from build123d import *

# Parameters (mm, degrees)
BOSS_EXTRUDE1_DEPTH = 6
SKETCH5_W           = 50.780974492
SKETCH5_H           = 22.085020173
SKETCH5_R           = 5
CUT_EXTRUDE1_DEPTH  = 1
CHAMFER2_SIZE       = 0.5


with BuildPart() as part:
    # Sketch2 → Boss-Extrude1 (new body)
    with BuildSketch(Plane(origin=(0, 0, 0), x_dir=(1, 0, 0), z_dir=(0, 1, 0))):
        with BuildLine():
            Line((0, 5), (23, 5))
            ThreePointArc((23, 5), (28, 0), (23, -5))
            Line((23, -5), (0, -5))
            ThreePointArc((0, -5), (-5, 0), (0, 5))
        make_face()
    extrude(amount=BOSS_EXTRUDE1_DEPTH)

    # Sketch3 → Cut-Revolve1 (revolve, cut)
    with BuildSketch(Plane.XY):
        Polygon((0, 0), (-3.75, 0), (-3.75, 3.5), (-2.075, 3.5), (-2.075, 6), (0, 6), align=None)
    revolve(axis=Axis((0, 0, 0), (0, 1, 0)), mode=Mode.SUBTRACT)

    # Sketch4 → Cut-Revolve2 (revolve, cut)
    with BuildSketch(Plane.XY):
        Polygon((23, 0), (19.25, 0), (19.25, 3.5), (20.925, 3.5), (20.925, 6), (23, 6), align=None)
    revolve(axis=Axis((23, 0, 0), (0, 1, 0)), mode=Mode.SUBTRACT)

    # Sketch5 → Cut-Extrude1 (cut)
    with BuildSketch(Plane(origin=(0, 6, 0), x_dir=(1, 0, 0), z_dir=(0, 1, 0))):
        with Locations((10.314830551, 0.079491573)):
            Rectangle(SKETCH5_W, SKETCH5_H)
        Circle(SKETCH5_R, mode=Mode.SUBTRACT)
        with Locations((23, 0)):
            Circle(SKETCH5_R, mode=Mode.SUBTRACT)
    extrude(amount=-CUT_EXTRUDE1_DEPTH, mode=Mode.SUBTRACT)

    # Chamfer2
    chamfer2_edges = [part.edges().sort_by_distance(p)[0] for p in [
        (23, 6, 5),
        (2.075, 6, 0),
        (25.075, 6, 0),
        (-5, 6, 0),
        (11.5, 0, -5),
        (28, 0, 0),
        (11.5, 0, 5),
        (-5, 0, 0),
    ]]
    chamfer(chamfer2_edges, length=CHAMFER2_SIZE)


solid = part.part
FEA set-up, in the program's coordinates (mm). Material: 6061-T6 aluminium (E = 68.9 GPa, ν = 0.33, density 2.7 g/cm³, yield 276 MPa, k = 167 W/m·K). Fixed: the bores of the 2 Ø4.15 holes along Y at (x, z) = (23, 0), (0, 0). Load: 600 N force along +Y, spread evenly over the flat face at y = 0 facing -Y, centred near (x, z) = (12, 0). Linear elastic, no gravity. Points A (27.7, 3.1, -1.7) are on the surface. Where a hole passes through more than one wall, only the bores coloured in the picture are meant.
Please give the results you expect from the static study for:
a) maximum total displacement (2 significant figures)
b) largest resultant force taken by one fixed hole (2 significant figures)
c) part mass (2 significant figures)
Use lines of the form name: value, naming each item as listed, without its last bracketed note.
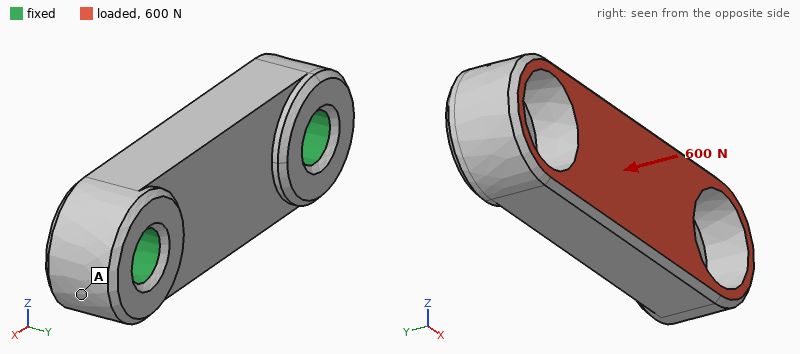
maximum total displacement: 5.4 µm
largest resultant force taken by one fixed hole: 370 N
part mass: 3.5 g
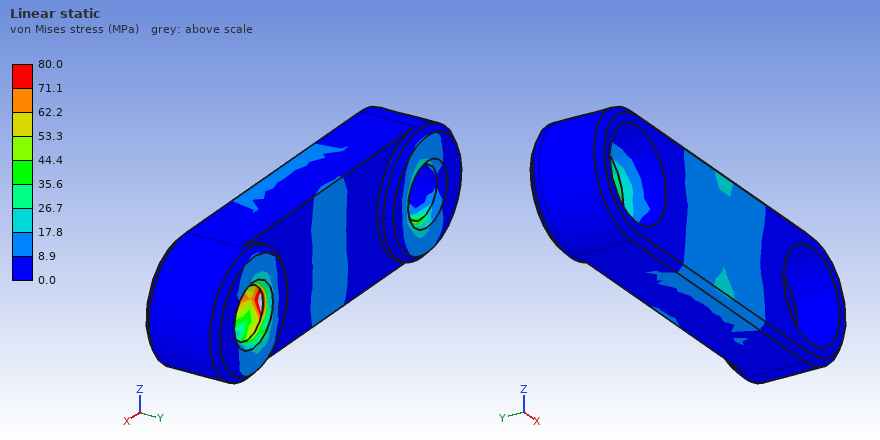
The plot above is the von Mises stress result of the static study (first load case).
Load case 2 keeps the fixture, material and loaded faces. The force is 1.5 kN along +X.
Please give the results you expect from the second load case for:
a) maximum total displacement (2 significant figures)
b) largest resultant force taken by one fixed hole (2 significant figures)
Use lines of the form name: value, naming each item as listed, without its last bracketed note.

maximum total displacement: 5.4 µm
largest resultant force taken by one fixed hole: 800 N
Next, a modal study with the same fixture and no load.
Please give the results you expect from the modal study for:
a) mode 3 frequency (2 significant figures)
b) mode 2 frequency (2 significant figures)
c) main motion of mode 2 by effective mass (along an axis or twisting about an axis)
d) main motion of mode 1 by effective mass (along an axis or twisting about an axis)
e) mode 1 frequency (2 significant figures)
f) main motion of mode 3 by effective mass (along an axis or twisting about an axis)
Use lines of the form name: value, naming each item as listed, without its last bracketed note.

mode 3 frequency: 51 kHz
mode 2 frequency: 35 kHz
main motion of mode 2 by effective mass: along Y
main motion of mode 1 by effective mass: along Z
mode 1 frequency: 30 kHz
main motion of mode 3 by effective mass: along Z
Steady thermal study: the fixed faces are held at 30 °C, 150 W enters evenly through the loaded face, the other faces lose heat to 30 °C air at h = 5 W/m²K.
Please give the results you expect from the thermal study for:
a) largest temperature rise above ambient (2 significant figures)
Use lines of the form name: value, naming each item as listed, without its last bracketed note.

largest temperature rise above ambient: 86 K
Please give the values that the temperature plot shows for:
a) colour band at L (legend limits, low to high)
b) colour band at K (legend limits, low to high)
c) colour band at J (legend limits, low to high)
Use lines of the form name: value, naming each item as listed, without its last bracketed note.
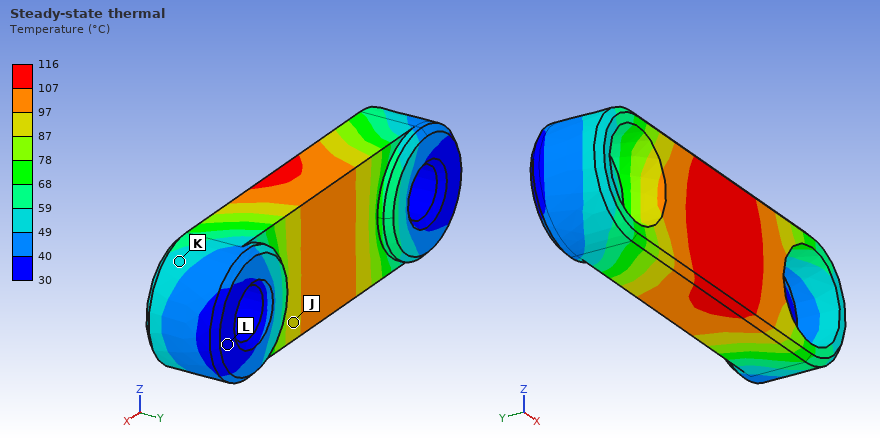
colour band at L: 30 to 40 °C
colour band at K: 49 to 59 °C
colour band at J: 87 to 97 °C
